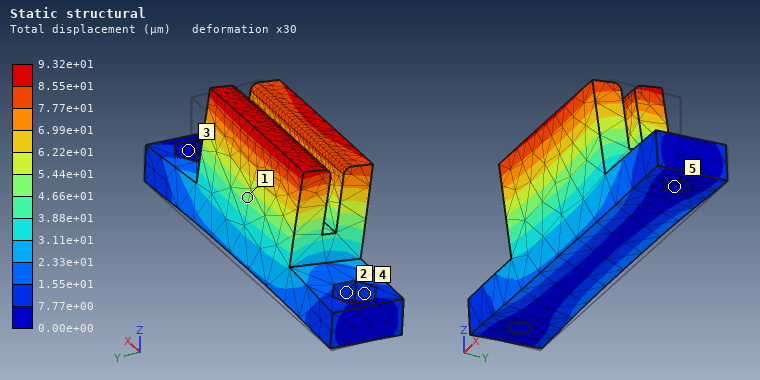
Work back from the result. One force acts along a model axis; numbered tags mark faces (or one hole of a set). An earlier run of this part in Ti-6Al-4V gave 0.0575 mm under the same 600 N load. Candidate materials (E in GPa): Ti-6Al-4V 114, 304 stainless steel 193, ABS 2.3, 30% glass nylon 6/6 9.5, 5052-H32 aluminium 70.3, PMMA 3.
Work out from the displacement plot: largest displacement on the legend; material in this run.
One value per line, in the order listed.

9.32e+01 µm
5052-H32 aluminium
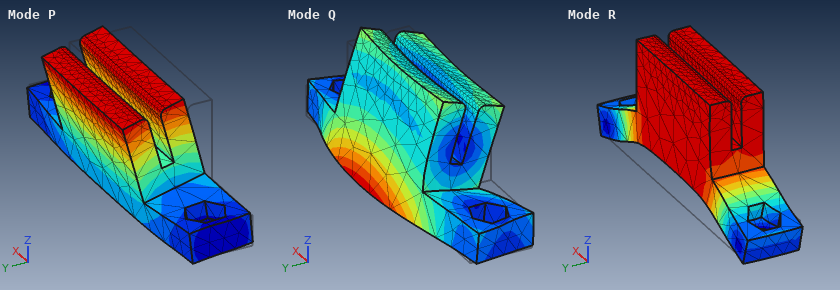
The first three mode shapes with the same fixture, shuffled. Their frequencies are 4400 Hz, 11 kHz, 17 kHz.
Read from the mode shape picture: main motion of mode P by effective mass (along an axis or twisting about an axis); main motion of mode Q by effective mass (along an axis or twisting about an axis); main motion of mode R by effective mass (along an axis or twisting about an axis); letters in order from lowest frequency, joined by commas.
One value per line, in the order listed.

along Y
along Y
along Z
P, R, Q
